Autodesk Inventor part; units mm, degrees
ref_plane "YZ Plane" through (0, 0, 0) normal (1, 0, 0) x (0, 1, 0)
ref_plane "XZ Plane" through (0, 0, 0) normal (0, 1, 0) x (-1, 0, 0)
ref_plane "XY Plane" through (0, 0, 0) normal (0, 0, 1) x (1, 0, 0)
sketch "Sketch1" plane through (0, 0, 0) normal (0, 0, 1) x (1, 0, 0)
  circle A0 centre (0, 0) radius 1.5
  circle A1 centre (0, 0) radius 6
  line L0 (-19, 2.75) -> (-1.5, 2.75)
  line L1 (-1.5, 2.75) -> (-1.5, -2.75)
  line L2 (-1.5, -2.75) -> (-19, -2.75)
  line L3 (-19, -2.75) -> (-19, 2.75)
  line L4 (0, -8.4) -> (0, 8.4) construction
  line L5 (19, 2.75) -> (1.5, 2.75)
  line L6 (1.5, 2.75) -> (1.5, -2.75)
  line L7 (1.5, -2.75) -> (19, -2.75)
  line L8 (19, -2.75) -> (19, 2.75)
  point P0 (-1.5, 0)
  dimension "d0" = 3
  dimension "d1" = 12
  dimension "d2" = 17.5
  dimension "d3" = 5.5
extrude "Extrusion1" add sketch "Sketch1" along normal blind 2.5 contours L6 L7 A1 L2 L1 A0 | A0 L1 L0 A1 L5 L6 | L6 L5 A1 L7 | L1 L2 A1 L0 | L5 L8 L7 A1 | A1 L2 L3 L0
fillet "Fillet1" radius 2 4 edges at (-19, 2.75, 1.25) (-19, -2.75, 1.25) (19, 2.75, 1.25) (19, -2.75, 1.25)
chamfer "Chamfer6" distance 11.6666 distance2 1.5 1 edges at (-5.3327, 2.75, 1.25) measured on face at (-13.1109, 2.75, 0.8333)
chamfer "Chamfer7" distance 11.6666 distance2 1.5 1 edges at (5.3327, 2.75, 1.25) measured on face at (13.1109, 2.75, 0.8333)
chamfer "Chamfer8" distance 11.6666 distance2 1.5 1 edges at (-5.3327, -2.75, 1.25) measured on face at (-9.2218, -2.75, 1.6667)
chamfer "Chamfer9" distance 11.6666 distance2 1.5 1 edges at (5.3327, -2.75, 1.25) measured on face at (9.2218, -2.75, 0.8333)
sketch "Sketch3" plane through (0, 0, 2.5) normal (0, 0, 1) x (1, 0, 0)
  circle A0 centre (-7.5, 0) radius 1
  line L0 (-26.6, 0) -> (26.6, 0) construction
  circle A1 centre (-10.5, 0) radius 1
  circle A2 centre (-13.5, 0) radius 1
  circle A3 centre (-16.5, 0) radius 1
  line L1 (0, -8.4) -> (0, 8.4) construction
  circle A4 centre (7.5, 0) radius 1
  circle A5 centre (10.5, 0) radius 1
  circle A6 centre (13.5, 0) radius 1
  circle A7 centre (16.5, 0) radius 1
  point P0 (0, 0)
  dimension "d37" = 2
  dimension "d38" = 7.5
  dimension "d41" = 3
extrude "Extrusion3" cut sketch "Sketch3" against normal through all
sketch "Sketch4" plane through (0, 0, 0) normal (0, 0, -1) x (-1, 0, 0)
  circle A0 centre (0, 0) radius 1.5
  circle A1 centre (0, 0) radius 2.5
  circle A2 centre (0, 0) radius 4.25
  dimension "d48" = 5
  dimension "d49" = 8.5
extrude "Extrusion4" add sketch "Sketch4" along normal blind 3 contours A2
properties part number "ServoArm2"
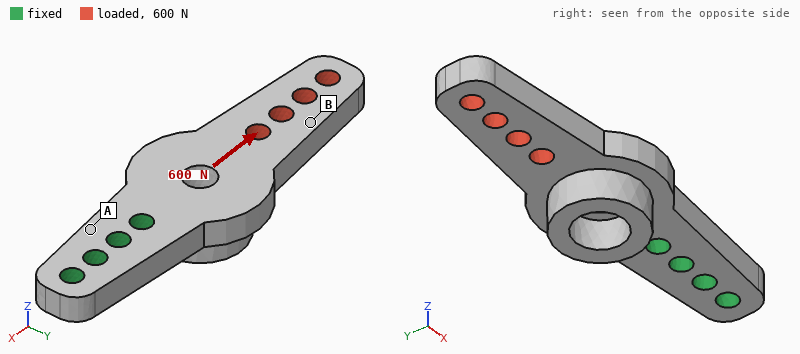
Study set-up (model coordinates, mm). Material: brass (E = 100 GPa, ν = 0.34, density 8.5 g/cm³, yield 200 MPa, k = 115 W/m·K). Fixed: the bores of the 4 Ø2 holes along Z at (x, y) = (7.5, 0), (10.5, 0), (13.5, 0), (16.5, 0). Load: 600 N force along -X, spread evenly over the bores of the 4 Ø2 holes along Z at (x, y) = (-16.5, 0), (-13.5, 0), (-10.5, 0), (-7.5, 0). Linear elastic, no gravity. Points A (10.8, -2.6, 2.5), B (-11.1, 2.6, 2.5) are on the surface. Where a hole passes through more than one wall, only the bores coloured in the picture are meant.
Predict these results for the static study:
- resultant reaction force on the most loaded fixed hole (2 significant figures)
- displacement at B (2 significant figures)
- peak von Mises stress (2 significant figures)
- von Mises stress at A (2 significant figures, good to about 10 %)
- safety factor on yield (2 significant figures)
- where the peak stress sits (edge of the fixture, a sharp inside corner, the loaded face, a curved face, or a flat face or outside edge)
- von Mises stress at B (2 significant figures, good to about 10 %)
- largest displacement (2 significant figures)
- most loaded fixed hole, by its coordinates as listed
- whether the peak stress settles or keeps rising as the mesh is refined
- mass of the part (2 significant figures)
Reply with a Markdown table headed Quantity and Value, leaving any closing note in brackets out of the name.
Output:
| Quantity | Value |
|---|---|
| resultant reaction force on the most loaded fixed hole | 450 N |
| displacement at B | 9.5 µm |
| peak von Mises stress | 93 MPa |
| von Mises stress at A | 8.6 MPa |
| safety factor on yield | 2.2 |
| where the peak stress sits | a curved face |
| von Mises stress at B | 27 MPa |
| largest displacement | 14 µm |
| most loaded fixed hole, by its coordinates as listed | (7.5, 0) |
| whether the peak stress settles or keeps rising as the mesh is refined | settles |
| mass of the part | 6.3 g |
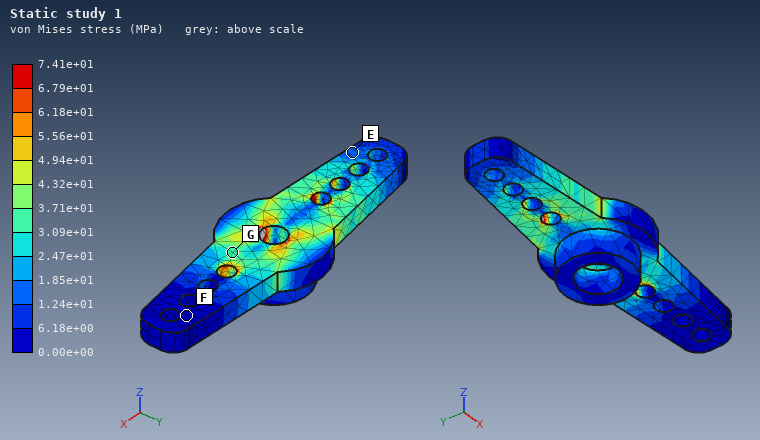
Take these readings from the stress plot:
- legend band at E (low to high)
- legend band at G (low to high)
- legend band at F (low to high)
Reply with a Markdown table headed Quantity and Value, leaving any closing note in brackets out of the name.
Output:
| Quantity | Value |
|---|---|
| legend band at E | 1.24e+01 to 1.85e+01 MPa |
| legend band at G | 3.09e+01 to 3.71e+01 MPa |
| legend band at F | 0.00e+00 to 6.18e+00 MPa |
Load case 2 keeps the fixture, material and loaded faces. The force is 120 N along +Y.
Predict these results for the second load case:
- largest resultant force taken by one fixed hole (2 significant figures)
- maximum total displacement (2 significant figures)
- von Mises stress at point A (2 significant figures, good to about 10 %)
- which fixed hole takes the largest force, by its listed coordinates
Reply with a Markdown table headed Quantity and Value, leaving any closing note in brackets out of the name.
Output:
| Quantity | Value |
|---|---|
| largest resultant force taken by one fixed hole | 400 N |
| maximum total displacement | 61 µm |
| von Mises stress at point A | 27 MPa |
| which fixed hole takes the largest force, by its listed coordinates | (7.5, 0) |
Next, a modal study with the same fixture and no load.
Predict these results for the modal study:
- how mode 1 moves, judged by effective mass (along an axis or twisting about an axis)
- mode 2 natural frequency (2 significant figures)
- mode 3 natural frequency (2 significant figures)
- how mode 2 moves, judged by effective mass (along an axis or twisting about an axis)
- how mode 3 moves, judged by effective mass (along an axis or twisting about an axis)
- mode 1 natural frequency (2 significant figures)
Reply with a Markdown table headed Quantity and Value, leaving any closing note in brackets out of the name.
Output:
| Quantity | Value |
|---|---|
| how mode 1 moves, judged by effective mass | along Z |
| mode 2 natural frequency | 6000 Hz |
| mode 3 natural frequency | 11 kHz |
| how mode 2 moves, judged by effective mass | along Y |
| how mode 3 moves, judged by effective mass | along Z |
| mode 1 natural frequency | 2700 Hz |
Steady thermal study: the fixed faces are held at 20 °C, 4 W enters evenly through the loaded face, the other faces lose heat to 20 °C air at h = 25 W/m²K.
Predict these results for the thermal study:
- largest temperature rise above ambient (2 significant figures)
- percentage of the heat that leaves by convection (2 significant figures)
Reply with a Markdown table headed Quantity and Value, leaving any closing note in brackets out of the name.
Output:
| Quantity | Value |
|---|---|
| largest temperature rise above ambient | 34 K |
| percentage of the heat that leaves by convection | 6.8 % |
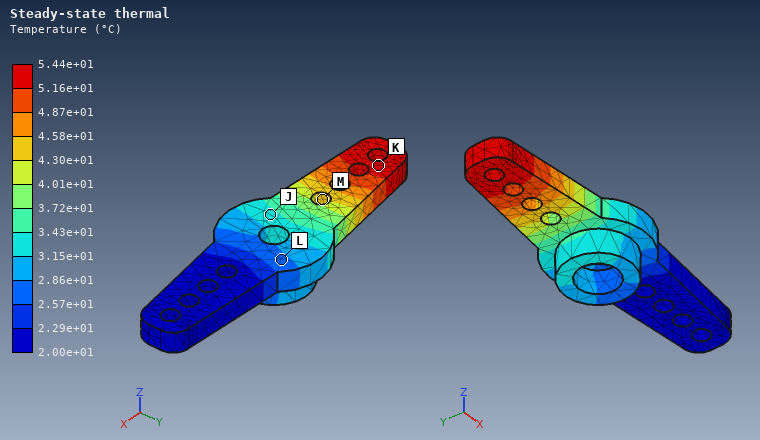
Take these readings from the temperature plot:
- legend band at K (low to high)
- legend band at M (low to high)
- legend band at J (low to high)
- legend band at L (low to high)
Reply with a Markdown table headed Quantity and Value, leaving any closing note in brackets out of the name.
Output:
| Quantity | Value |
|---|---|
| legend band at K | 5.16e+01 to 5.44e+01 °C |
| legend band at M | 4.30e+01 to 4.58e+01 °C |
| legend band at J | 3.15e+01 to 3.43e+01 °C |
| legend band at L | 2.57e+01 to 2.86e+01 °C |
